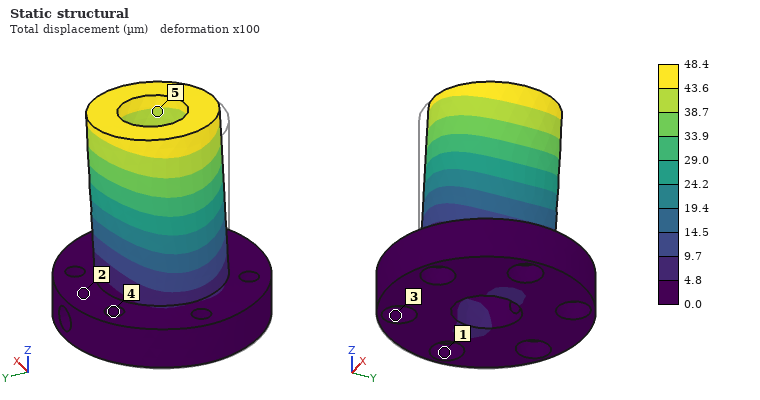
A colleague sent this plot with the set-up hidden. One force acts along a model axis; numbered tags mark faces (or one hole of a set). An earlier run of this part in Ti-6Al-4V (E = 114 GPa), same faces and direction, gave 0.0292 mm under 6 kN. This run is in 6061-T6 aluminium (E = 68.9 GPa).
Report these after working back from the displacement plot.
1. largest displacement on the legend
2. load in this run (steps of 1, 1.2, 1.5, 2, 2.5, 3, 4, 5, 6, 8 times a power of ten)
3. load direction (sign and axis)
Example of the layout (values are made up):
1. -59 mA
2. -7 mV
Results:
1. 48.4 µm
2. 6 kN
3. +X
